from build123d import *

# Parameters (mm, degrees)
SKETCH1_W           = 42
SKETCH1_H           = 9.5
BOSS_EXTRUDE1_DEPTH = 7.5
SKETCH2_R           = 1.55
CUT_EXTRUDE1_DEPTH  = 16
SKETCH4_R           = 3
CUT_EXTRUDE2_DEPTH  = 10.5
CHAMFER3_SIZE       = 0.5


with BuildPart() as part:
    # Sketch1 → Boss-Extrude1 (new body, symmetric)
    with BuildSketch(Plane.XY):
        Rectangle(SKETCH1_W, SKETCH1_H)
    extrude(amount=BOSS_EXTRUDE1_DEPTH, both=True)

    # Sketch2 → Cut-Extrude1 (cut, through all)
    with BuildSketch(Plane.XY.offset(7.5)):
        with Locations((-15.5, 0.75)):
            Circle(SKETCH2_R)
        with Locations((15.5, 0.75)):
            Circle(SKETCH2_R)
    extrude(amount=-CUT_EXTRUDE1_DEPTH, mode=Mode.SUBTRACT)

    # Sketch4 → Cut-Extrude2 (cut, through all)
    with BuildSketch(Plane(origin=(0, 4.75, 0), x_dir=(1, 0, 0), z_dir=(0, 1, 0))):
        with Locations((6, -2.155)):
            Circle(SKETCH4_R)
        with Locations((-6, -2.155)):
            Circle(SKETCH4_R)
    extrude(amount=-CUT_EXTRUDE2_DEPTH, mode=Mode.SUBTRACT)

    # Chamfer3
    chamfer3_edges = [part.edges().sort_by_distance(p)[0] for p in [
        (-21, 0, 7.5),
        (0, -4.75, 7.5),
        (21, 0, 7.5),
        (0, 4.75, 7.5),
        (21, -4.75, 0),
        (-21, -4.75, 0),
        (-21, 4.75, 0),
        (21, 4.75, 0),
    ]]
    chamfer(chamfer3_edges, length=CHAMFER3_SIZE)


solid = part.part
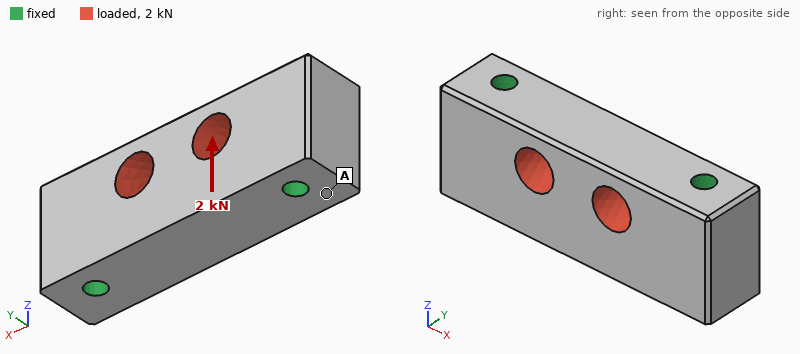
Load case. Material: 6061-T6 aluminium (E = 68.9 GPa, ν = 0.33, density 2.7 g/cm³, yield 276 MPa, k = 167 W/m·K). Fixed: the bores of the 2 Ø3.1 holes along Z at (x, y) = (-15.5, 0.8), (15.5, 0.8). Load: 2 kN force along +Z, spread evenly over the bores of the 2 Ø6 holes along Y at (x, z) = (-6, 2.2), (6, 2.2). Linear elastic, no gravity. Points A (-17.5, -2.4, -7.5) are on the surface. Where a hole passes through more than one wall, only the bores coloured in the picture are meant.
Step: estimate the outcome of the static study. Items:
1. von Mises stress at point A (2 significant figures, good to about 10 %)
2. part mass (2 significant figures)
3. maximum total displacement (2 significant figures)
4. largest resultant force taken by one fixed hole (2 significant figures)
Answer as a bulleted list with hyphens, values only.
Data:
- 6.8 MPa
- 14 g
- 6.1 µm
- 1.0 kN
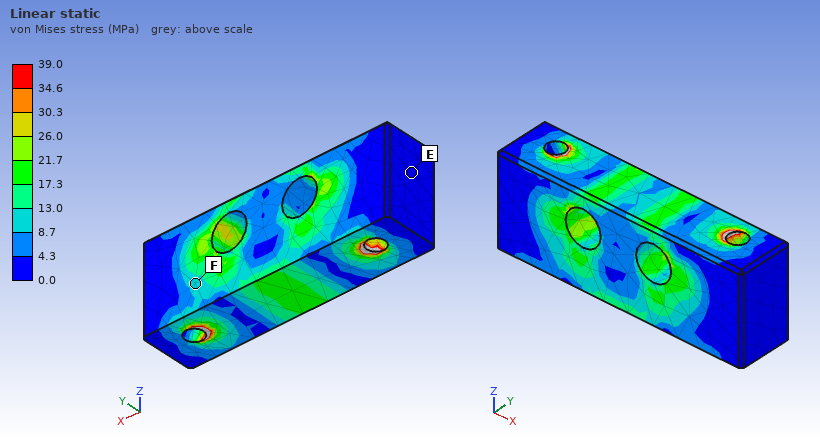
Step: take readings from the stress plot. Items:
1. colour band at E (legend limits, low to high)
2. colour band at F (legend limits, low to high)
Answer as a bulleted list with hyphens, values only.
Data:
- 0.0 to 4.3 MPa
- 8.7 to 13.0 MPa
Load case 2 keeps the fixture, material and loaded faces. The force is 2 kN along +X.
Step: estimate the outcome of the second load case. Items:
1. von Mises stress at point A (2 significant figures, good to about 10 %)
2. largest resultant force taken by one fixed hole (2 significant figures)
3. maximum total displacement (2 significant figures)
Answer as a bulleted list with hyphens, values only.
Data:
- 2.9 MPa
- 1.0 kN
- 2.4 µm
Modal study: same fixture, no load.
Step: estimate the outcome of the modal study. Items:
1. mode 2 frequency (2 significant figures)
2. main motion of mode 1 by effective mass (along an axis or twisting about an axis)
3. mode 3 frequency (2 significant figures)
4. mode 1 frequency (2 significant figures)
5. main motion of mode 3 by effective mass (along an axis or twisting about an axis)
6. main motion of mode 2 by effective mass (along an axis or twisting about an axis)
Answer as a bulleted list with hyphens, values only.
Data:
- 37 kHz
- along Y
- 42 kHz
- 30 kHz
- twisting about X
- along Z
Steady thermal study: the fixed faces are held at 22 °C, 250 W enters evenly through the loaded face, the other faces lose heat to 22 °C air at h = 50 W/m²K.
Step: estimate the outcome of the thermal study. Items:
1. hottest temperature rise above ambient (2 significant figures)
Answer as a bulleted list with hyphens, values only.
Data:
- 74 K
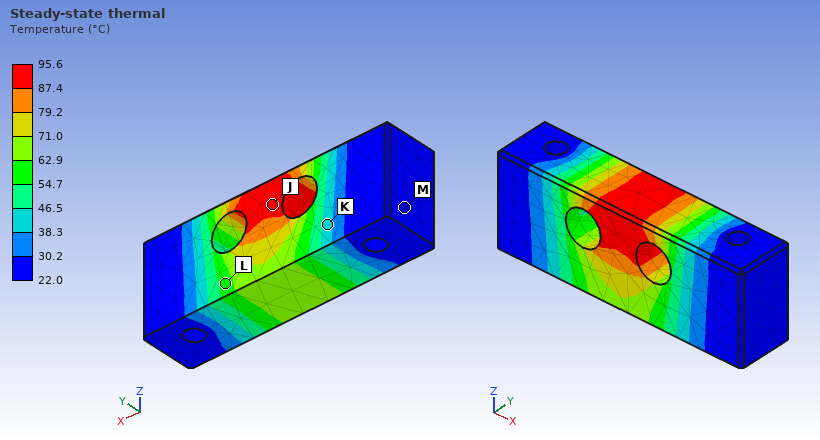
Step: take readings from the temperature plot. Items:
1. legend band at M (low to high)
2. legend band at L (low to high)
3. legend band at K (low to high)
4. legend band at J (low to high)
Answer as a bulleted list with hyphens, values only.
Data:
- 22.0 to 30.2 °C
- 54.7 to 62.9 °C
- 38.3 to 46.5 °C
- 87.4 to 95.6 °C
